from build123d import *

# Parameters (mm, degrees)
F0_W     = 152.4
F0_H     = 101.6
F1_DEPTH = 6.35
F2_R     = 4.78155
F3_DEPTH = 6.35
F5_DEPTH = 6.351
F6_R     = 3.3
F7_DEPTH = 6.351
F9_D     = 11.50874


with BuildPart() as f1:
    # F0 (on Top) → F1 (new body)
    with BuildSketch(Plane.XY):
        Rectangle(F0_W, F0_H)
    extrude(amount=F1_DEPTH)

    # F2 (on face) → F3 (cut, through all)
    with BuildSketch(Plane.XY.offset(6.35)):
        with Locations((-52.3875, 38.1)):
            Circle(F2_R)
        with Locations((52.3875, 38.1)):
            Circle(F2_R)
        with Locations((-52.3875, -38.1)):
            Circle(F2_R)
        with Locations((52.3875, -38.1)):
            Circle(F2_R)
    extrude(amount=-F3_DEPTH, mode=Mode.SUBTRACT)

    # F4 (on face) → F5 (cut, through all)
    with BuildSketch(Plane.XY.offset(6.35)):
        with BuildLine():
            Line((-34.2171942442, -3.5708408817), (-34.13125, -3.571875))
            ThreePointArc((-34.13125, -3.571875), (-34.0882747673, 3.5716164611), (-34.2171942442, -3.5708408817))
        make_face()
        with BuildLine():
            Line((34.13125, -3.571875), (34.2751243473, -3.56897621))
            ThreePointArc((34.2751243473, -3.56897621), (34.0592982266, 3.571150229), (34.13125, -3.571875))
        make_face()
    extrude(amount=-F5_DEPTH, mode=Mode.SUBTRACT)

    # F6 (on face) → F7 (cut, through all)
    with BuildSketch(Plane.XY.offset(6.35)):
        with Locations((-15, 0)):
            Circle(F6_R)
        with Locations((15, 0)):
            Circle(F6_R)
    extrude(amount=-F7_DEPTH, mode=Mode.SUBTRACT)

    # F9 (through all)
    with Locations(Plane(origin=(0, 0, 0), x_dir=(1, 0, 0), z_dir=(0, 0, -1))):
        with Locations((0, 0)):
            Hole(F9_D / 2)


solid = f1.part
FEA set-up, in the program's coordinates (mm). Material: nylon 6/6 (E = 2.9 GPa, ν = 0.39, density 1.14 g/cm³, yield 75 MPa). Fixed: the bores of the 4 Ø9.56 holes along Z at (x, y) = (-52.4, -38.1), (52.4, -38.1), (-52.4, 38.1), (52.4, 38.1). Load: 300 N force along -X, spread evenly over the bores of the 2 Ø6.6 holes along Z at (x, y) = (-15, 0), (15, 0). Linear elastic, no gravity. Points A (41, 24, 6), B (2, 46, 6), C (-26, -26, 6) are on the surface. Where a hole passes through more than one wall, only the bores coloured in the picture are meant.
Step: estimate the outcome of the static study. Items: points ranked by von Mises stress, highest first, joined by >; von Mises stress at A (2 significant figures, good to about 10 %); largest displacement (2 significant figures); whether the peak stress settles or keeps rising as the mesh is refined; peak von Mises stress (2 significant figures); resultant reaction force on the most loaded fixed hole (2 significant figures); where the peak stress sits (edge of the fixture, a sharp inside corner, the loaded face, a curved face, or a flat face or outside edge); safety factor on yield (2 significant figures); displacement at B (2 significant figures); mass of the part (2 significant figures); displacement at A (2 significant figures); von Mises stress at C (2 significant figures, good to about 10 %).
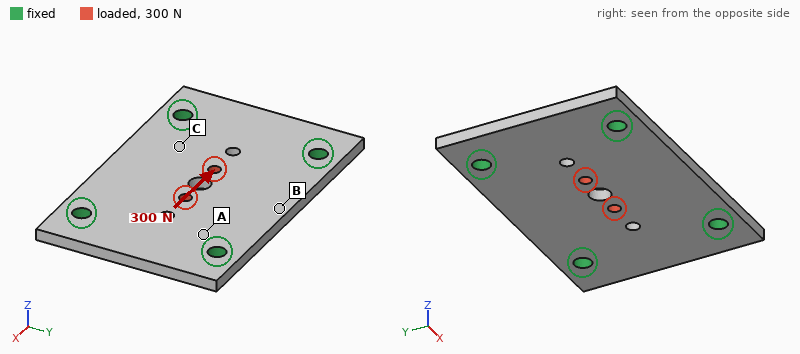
A > C > B
0.45 MPa
13 µm
settles
2.1 MPa
79 N
the loaded face
36
2.3 µm
110 g
3.1 µm
0.32 MPa
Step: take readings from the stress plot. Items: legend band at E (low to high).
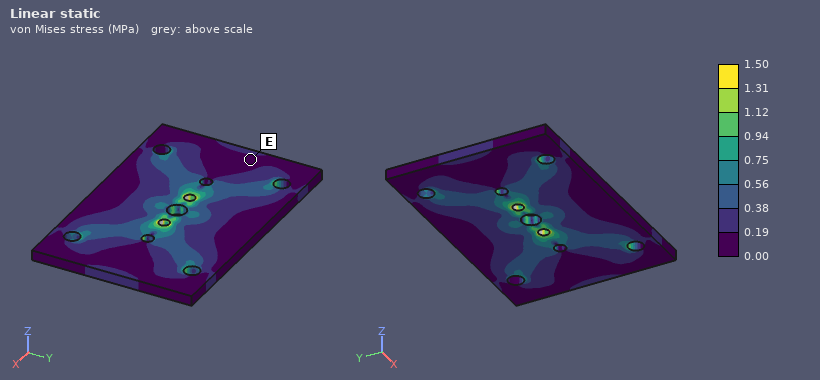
0.00 to 0.19 MPa
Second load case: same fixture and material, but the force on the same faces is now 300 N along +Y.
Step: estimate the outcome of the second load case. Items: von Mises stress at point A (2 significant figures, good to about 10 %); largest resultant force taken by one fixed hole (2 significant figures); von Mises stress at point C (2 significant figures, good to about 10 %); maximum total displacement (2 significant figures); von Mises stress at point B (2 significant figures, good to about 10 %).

0.57 MPa
89 N
0.48 MPa
15 µm
0.26 MPa
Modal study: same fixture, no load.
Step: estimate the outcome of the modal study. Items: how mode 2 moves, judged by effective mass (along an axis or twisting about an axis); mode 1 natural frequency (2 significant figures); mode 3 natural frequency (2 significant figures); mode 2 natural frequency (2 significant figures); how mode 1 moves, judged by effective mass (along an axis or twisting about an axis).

twisting about X
880 Hz
1600 Hz
1200 Hz
along Z
